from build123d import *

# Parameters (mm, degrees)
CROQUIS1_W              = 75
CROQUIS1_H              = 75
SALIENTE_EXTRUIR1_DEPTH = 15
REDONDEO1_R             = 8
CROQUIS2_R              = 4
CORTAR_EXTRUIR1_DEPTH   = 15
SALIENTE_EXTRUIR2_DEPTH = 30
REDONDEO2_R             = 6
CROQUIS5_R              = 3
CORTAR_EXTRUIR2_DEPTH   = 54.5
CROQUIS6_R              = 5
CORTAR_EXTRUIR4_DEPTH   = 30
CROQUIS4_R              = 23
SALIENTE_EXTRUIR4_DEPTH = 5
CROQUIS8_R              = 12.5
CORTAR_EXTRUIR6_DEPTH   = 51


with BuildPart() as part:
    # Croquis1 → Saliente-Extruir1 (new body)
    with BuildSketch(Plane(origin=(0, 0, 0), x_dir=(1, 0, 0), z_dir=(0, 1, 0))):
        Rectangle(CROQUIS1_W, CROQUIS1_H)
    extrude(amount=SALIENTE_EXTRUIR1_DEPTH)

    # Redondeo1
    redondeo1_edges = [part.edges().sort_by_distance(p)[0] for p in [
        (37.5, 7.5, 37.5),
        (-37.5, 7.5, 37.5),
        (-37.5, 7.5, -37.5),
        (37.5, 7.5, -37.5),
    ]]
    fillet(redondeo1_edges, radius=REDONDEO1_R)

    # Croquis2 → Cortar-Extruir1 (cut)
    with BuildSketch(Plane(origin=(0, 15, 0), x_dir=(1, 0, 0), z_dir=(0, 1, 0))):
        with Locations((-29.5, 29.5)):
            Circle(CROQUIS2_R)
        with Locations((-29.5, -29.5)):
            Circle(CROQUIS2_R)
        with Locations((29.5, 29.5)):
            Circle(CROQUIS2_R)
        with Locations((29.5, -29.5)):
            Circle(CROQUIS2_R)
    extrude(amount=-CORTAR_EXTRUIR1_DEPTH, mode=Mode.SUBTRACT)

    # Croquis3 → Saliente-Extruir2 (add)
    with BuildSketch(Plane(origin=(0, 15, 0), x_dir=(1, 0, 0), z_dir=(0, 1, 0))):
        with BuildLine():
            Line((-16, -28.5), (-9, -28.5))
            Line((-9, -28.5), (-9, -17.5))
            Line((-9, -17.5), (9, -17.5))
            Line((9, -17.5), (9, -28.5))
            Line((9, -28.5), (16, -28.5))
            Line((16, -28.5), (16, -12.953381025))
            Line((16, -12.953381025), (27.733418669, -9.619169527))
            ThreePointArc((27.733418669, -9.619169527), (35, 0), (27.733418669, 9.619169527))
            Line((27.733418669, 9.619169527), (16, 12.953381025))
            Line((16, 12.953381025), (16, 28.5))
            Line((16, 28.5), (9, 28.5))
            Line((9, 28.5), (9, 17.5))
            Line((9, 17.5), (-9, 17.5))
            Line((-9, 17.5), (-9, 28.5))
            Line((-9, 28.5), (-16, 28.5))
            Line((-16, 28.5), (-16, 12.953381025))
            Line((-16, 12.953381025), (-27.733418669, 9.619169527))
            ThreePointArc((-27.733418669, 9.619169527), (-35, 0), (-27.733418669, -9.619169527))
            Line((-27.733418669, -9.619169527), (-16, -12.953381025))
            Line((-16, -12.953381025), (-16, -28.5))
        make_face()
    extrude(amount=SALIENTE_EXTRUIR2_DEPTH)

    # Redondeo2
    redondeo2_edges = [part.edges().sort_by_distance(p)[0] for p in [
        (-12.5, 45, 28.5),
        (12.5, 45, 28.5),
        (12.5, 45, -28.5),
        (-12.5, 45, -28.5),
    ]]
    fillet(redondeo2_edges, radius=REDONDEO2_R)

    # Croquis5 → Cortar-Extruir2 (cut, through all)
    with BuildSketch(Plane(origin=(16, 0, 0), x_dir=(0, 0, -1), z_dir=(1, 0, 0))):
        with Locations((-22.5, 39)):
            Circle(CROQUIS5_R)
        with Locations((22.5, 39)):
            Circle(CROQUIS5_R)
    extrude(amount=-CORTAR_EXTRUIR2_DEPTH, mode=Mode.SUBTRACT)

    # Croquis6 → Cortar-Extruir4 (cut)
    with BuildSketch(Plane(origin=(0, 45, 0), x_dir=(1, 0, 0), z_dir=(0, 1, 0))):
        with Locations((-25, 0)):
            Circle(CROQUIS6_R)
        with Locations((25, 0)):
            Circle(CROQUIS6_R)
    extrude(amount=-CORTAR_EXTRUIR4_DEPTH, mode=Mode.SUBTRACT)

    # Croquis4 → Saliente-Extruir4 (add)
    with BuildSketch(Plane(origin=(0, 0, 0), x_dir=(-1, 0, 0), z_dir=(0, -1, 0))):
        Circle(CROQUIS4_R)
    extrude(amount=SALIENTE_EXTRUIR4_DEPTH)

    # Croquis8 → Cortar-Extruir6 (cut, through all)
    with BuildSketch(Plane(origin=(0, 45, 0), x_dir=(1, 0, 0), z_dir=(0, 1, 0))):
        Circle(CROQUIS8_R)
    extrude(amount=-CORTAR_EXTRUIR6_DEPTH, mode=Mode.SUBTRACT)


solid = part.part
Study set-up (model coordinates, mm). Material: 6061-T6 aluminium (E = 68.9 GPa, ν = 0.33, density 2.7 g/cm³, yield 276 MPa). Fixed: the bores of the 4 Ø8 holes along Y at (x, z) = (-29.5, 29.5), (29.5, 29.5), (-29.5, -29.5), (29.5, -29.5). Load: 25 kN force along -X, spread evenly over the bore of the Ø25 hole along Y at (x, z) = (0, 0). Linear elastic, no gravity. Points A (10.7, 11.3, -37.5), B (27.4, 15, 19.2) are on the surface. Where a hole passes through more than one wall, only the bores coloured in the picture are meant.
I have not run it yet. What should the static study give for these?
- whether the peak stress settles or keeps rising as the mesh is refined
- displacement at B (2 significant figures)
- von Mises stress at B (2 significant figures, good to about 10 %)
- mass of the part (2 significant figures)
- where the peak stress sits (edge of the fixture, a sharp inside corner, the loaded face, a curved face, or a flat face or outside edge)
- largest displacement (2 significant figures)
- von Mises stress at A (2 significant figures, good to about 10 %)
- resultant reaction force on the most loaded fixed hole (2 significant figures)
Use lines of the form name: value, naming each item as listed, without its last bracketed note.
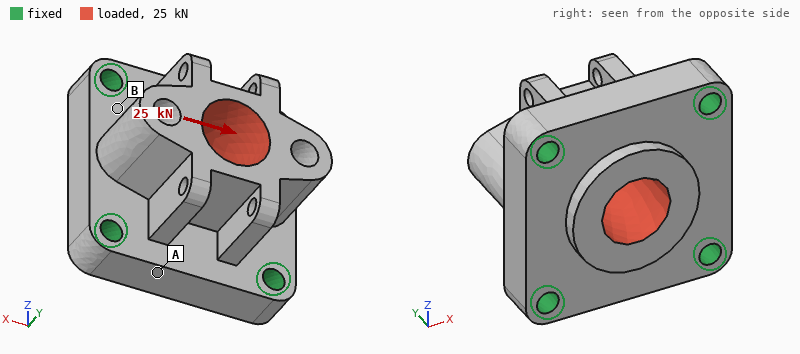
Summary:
whether the peak stress settles or keeps rising as the mesh is refined: keeps rising
displacement at B: 7.1 µm
von Mises stress at B: 29 MPa
mass of the part: 330 g
where the peak stress sits: edge of the fixture
largest displacement: 38 µm
von Mises stress at A: 8.0 MPa
resultant reaction force on the most loaded fixed hole: 7.4 kN
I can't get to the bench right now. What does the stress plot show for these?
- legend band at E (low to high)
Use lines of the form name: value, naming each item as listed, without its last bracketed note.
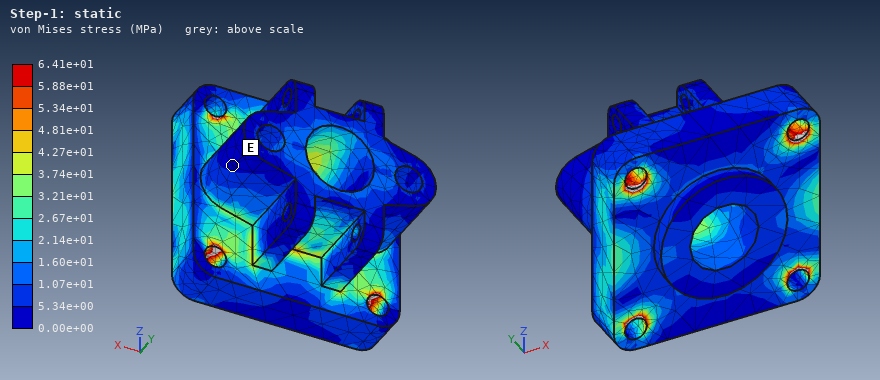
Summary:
legend band at E: 0.00e+00 to 5.34e+00 MPa
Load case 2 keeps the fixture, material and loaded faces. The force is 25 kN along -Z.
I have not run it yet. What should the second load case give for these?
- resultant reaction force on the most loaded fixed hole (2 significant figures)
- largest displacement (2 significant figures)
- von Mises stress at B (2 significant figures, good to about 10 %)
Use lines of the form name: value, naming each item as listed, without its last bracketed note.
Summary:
resultant reaction force on the most loaded fixed hole: 7.4 kN
largest displacement: 37 µm
von Mises stress at B: 29 MPa
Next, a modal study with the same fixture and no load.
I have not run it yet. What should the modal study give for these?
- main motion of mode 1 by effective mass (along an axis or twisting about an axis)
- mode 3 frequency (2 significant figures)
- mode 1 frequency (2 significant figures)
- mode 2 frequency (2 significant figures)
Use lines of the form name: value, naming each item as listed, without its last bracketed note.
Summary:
main motion of mode 1 by effective mass: along X
mode 3 frequency: 11 kHz
mode 1 frequency: 10 kHz
mode 2 frequency: 11 kHz
